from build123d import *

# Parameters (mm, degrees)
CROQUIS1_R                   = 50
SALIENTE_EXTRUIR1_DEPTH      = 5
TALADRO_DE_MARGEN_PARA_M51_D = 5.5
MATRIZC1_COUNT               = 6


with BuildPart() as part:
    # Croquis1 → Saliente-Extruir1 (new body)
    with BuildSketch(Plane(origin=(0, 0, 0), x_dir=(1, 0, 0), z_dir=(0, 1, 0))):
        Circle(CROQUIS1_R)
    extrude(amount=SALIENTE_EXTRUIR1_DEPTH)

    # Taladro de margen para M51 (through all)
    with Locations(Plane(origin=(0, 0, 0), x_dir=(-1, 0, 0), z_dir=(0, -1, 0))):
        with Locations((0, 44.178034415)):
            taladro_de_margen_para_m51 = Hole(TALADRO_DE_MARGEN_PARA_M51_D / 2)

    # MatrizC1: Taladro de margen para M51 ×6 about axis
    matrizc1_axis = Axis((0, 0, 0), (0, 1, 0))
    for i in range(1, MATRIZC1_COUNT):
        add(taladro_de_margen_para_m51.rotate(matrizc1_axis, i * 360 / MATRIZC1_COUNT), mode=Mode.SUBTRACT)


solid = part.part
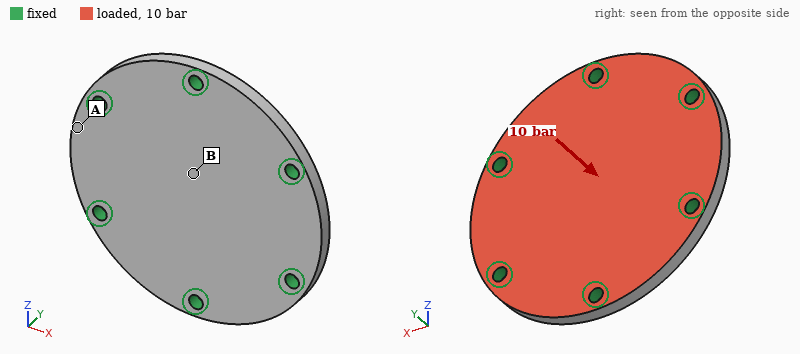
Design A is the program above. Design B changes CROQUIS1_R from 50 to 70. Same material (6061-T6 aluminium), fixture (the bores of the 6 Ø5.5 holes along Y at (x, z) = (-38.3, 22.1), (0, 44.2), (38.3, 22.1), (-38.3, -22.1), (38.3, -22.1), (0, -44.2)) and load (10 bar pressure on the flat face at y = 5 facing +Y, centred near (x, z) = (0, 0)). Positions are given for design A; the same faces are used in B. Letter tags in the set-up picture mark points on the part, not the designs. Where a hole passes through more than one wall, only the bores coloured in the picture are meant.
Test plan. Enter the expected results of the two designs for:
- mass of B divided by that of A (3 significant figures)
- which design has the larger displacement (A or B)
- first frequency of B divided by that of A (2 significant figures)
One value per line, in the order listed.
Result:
1.98
B
0.81
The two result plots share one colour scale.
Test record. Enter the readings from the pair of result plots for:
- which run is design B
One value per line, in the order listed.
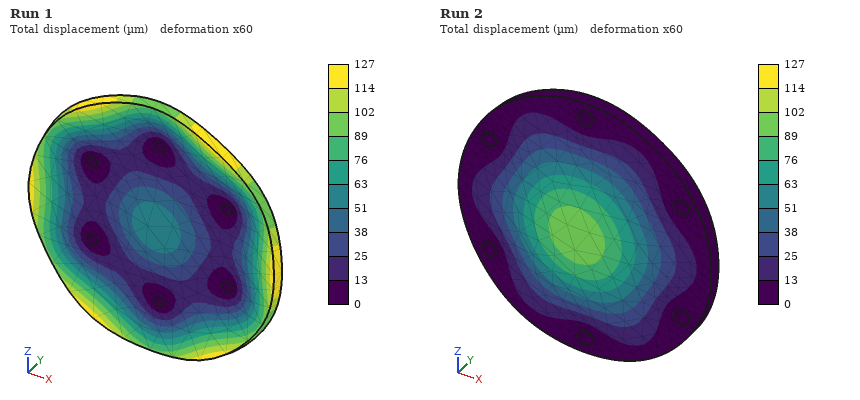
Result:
Run 1
